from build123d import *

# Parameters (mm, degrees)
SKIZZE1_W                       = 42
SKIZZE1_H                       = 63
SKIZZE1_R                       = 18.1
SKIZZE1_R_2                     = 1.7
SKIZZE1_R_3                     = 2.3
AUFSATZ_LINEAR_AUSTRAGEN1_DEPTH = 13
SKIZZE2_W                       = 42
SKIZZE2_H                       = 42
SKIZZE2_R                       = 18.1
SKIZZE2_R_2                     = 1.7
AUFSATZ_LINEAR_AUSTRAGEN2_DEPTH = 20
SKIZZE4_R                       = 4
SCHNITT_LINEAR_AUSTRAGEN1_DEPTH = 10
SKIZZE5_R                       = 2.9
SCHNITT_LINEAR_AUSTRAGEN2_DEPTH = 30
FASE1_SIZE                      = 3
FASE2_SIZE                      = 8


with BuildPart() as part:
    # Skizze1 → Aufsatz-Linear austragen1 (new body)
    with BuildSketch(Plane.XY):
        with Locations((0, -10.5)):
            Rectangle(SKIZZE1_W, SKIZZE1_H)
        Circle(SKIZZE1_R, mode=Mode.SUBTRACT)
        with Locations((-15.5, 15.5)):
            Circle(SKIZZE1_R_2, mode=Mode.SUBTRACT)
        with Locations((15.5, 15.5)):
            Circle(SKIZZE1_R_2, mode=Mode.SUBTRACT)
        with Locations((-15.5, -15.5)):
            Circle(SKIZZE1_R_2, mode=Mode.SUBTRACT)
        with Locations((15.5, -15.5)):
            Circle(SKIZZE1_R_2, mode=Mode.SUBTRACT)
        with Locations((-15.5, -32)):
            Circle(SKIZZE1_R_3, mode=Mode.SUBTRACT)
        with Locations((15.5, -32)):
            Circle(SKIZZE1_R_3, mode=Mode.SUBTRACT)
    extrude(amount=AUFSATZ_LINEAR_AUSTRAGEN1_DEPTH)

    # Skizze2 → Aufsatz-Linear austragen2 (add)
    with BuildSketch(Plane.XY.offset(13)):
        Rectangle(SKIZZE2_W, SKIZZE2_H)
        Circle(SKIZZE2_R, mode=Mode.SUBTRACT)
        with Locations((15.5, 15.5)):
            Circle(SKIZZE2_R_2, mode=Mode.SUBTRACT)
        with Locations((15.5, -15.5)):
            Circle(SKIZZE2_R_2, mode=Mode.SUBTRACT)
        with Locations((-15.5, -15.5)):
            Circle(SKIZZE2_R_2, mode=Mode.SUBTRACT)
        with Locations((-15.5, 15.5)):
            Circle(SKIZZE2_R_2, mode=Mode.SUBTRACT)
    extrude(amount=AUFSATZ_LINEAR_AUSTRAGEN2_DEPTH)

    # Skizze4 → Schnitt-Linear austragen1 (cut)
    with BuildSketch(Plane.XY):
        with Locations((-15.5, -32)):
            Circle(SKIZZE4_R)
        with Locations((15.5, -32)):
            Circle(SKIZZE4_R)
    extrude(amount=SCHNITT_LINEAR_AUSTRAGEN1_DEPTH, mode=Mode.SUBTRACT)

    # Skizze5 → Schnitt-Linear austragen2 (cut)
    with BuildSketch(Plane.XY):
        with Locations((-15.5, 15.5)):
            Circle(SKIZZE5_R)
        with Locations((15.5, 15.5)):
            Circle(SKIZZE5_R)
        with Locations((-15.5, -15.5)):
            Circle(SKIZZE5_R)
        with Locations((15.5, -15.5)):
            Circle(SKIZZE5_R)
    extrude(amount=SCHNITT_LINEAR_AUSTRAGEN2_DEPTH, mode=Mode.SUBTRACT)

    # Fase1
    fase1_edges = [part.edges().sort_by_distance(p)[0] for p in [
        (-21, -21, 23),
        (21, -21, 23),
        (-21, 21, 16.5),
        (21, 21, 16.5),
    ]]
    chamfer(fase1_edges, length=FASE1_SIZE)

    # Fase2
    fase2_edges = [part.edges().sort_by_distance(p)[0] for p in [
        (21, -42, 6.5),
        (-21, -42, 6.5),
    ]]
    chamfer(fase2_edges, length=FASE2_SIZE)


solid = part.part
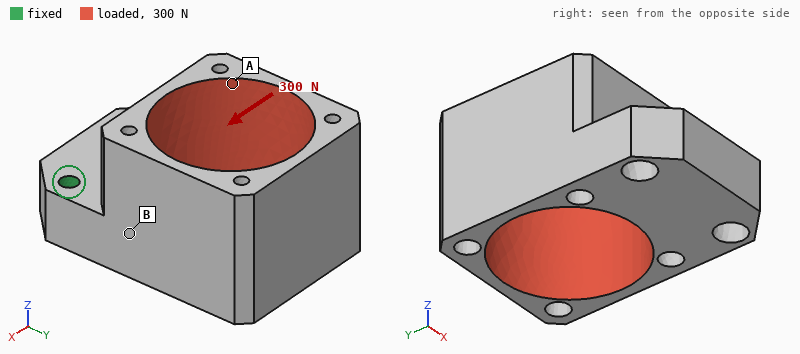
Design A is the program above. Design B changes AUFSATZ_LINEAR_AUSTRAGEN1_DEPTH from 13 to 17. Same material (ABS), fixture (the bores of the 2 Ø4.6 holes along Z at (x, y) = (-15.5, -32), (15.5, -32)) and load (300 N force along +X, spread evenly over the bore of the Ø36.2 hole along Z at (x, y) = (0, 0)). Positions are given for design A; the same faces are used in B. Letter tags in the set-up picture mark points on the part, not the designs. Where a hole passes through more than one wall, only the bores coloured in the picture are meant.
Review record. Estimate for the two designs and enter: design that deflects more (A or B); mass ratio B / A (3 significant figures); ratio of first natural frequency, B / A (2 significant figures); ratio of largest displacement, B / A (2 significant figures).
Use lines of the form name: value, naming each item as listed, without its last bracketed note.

design that deflects more: A
mass ratio B / A: 1.11
ratio of first natural frequency, B / A: 1.8
ratio of largest displacement, B / A: 0.77
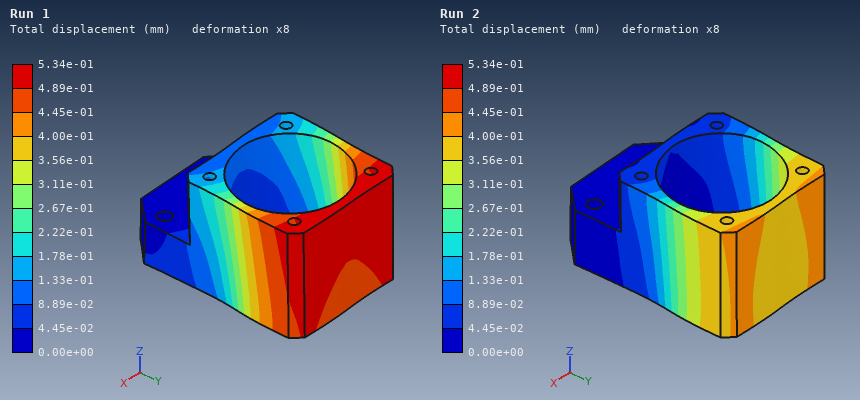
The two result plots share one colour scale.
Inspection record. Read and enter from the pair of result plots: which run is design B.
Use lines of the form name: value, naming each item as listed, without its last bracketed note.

which run is design B: Run 2
